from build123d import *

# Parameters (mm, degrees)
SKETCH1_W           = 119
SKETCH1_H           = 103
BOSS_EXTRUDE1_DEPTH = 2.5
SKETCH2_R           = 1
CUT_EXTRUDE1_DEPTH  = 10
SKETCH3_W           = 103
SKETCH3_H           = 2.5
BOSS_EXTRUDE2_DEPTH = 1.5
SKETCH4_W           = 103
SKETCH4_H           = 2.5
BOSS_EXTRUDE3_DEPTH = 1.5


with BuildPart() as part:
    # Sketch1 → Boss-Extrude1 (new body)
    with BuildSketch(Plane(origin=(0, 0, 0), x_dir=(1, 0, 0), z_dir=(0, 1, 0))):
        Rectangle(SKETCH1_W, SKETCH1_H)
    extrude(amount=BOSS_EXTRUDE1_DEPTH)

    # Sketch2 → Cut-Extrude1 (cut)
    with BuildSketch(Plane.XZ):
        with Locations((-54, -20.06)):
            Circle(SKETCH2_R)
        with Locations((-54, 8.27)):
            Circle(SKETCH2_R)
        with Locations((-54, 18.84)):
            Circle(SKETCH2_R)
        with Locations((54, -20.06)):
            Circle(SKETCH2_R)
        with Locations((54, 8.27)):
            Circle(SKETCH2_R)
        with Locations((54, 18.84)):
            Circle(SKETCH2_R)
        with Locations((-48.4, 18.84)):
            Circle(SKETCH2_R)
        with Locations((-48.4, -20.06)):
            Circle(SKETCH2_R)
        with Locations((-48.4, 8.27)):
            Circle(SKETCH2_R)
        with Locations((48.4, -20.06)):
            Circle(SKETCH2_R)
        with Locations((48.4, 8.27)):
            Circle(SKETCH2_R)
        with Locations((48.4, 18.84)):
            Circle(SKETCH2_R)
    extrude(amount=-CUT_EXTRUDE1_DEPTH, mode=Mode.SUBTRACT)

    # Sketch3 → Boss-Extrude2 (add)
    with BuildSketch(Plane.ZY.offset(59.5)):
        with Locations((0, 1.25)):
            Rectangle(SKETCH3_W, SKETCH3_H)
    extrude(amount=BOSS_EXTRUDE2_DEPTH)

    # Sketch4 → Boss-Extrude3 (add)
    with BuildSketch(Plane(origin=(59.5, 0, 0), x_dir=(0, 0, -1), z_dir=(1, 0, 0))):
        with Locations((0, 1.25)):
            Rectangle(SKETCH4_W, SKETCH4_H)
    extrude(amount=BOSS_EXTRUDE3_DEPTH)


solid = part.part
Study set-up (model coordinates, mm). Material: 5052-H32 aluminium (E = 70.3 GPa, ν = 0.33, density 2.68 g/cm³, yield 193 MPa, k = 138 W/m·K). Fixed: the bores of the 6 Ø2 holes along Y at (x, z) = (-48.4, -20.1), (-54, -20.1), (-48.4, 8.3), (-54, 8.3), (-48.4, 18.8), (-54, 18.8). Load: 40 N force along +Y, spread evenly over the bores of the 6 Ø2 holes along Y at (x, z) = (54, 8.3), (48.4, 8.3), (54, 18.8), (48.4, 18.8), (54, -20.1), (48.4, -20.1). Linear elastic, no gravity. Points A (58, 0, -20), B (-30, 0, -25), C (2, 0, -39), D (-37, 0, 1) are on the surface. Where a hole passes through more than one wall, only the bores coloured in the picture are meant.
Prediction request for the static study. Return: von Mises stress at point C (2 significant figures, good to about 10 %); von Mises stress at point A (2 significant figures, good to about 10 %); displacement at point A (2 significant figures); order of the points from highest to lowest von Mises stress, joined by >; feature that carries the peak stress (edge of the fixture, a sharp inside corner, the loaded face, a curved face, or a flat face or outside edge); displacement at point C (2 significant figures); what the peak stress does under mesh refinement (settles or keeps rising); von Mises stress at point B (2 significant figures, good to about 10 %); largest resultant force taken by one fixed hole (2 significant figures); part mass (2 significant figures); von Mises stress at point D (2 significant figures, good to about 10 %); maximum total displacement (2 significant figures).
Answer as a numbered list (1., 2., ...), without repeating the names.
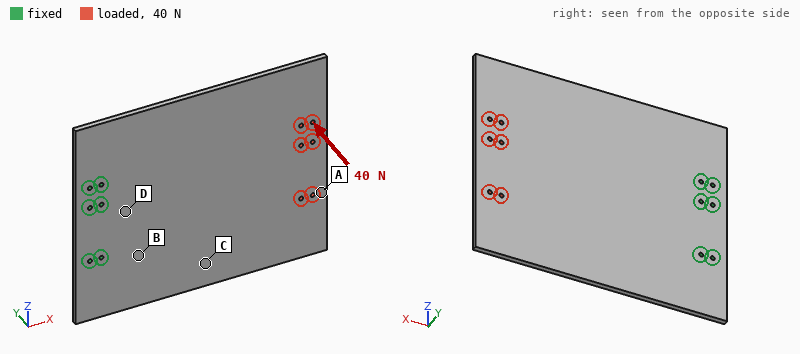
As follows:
1. 18 MPa
2. 6.0 MPa
3. 1.7 mm
4. D > B > C > A
5. edge of the fixture
6. 0.49 mm
7. keeps rising
8. 28 MPa
9. 160 N
10. 84 g
11. 35 MPa
12. 1.8 mm
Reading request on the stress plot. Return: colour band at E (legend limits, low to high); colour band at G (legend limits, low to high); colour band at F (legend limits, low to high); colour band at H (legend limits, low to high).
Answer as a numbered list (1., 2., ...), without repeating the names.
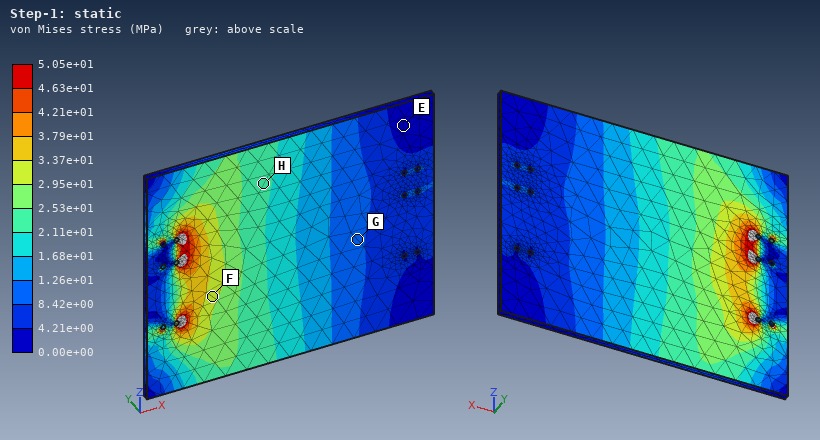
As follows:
1. 0.00e+00 to 4.21e+00 MPa
2. 8.42e+00 to 1.26e+01 MPa
3. 2.95e+01 to 3.37e+01 MPa
4. 2.11e+01 to 2.53e+01 MPa
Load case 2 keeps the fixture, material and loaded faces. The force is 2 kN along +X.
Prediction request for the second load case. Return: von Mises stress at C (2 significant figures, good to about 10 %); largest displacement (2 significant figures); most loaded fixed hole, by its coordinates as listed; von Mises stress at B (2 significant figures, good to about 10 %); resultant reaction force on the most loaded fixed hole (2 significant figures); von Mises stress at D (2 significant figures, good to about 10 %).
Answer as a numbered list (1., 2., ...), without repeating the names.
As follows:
1. 4.8 MPa
2. 21 µm
3. (-48.4, 18.8)
4. 9.4 MPa
5. 520 N
6. 10 MPa
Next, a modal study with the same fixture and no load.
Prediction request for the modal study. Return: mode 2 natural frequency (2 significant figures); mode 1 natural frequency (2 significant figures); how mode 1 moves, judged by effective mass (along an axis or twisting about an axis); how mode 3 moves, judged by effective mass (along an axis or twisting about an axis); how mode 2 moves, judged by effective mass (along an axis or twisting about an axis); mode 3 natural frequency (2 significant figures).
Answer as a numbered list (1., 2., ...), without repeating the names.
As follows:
1. 390 Hz
2. 170 Hz
3. along Y
4. along Y
5. twisting about X
6. 960 Hz
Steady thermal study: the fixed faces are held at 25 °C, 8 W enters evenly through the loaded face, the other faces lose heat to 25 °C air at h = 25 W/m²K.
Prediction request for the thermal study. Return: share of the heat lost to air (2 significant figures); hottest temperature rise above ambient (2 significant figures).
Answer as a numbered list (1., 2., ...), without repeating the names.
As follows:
1. 57 %
2. 18 K
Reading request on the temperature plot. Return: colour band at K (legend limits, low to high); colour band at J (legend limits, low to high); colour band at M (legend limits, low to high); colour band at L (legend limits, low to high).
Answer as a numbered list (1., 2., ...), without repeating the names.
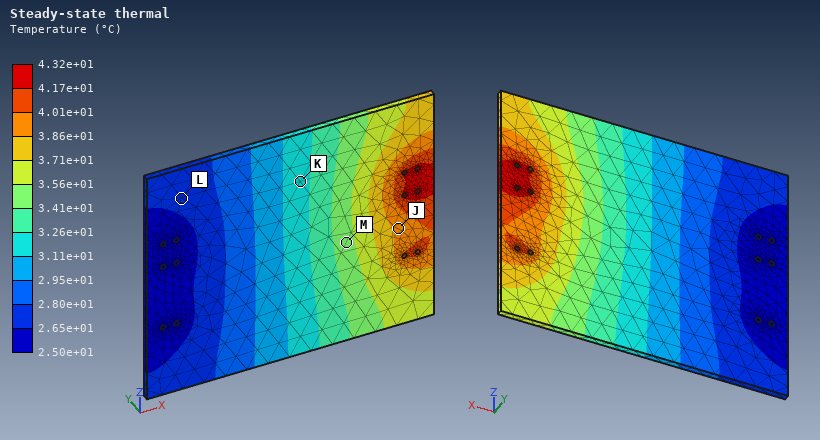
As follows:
1. 3.11e+01 to 3.26e+01 °C
2. 3.86e+01 to 4.01e+01 °C
3. 3.41e+01 to 3.56e+01 °C
4. 2.65e+01 to 2.80e+01 °C
